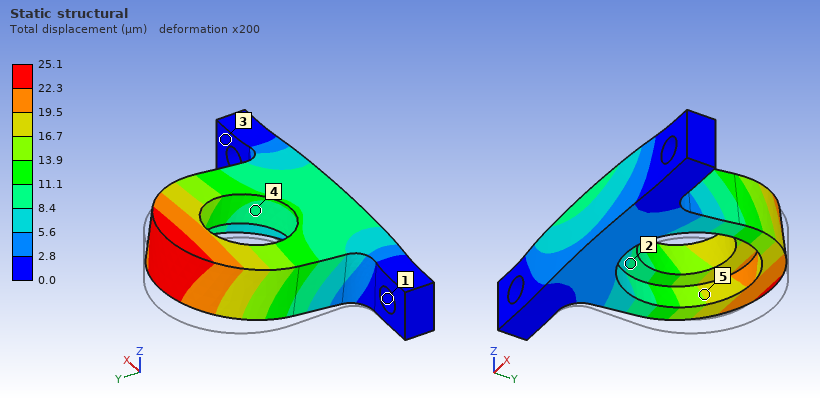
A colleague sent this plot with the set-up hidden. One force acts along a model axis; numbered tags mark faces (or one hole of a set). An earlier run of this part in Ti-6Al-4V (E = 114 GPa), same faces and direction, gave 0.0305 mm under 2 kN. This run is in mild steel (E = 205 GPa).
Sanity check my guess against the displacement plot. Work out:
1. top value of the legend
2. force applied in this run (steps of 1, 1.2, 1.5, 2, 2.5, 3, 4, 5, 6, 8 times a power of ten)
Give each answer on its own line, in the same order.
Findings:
25.1 µm
3 kN
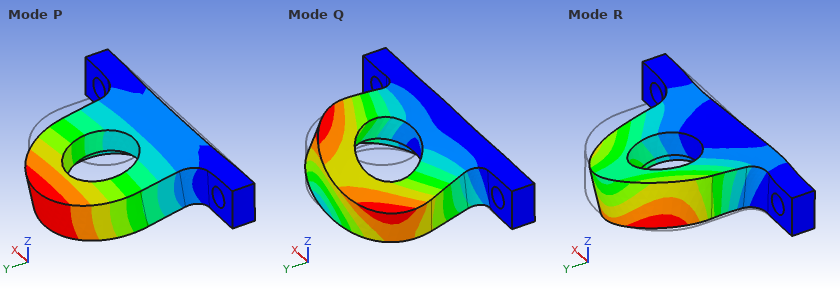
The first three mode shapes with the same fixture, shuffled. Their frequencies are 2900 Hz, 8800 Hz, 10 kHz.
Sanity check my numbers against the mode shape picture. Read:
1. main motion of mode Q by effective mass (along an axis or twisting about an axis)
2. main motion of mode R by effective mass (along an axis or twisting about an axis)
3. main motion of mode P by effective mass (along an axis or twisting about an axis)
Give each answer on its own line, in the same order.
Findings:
along X
along X
along Z
